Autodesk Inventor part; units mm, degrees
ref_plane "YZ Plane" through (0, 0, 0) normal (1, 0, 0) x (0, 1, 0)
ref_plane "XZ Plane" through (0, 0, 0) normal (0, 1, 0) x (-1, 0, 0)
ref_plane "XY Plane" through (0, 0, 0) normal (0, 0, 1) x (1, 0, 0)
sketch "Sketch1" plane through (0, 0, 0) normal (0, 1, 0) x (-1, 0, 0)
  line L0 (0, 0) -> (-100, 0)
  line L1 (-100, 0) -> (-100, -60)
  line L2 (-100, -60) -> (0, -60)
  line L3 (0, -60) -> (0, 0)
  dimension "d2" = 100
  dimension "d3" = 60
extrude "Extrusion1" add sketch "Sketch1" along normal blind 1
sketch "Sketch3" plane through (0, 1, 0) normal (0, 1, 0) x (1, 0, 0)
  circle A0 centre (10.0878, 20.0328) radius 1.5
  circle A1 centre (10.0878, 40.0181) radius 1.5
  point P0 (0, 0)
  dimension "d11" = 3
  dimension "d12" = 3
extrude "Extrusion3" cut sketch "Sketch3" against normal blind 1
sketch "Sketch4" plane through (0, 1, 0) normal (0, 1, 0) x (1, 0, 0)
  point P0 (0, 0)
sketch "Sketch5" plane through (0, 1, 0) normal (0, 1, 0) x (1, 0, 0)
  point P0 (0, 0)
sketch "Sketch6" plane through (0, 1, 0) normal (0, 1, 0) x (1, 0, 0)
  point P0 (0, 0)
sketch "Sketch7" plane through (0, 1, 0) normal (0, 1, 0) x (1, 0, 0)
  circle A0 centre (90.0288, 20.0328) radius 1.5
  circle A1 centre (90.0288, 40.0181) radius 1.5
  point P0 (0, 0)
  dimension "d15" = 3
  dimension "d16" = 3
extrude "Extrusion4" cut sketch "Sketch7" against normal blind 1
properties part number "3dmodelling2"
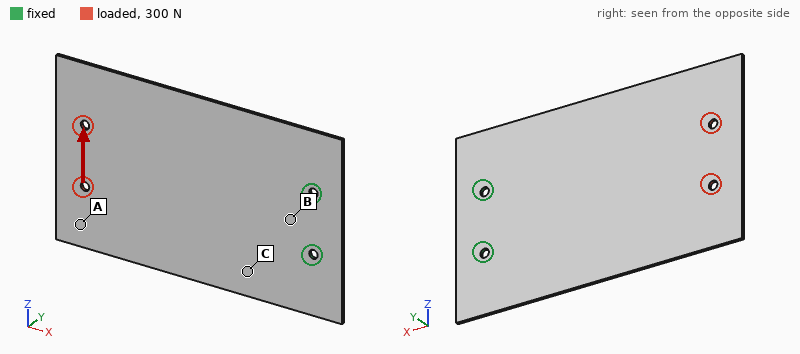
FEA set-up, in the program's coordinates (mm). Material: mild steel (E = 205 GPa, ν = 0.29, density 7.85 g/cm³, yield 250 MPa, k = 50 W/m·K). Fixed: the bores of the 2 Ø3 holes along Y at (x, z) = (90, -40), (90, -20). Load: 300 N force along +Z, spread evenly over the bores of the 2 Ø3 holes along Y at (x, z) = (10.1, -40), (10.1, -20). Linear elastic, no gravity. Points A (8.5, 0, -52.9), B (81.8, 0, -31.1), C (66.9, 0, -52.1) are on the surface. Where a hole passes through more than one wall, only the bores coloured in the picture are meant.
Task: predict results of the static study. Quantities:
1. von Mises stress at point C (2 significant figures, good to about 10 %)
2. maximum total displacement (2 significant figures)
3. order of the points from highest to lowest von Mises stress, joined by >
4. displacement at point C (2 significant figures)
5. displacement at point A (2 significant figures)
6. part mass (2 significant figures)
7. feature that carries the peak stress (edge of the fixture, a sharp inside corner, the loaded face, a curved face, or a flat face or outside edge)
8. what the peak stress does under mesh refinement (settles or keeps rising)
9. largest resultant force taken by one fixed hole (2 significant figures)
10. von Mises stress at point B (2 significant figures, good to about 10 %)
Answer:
21 MPa
63 µm
B > C > A
18 µm
56 µm
47 g
edge of the fixture
keeps rising
1.1 kN
47 MPa
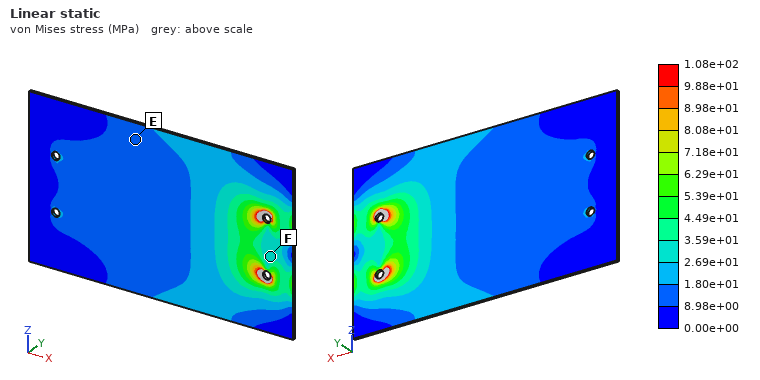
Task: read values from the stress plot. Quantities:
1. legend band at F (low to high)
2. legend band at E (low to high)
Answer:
2.69e+01 to 3.59e+01 MPa
8.98e+00 to 1.80e+01 MPa
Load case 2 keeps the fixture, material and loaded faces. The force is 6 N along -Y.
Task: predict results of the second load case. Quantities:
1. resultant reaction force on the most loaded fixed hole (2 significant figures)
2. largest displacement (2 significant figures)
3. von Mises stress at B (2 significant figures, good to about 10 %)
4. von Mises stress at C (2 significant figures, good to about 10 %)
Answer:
3.0 N
1.2 mm
46 MPa
33 MPa
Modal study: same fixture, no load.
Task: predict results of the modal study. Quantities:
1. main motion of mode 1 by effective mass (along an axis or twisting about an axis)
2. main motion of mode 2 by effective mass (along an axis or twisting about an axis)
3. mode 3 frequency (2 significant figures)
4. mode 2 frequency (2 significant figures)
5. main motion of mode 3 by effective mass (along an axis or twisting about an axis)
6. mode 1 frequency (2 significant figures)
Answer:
along Y
twisting about X
620 Hz
320 Hz
along Y
100 Hz
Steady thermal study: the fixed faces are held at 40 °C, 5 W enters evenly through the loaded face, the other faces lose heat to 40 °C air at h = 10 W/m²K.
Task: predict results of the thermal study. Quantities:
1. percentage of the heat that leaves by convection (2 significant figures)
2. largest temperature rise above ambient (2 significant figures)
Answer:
72 %
78 K
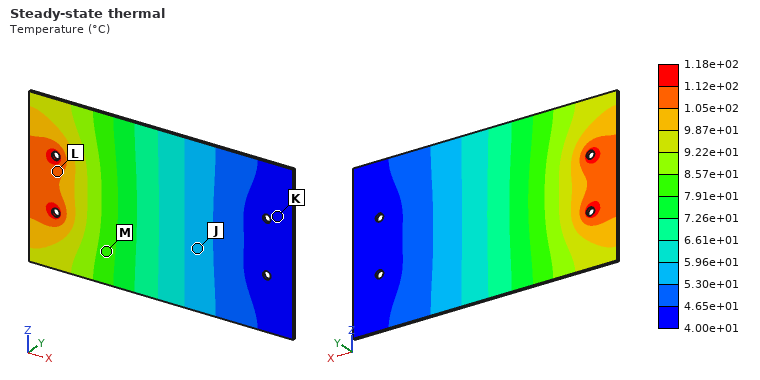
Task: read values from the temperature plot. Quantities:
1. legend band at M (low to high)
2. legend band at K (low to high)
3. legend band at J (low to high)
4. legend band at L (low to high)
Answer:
7.91e+01 to 8.57e+01 °C
4.00e+01 to 4.65e+01 °C
5.30e+01 to 5.96e+01 °C
1.05e+02 to 1.12e+02 °C
